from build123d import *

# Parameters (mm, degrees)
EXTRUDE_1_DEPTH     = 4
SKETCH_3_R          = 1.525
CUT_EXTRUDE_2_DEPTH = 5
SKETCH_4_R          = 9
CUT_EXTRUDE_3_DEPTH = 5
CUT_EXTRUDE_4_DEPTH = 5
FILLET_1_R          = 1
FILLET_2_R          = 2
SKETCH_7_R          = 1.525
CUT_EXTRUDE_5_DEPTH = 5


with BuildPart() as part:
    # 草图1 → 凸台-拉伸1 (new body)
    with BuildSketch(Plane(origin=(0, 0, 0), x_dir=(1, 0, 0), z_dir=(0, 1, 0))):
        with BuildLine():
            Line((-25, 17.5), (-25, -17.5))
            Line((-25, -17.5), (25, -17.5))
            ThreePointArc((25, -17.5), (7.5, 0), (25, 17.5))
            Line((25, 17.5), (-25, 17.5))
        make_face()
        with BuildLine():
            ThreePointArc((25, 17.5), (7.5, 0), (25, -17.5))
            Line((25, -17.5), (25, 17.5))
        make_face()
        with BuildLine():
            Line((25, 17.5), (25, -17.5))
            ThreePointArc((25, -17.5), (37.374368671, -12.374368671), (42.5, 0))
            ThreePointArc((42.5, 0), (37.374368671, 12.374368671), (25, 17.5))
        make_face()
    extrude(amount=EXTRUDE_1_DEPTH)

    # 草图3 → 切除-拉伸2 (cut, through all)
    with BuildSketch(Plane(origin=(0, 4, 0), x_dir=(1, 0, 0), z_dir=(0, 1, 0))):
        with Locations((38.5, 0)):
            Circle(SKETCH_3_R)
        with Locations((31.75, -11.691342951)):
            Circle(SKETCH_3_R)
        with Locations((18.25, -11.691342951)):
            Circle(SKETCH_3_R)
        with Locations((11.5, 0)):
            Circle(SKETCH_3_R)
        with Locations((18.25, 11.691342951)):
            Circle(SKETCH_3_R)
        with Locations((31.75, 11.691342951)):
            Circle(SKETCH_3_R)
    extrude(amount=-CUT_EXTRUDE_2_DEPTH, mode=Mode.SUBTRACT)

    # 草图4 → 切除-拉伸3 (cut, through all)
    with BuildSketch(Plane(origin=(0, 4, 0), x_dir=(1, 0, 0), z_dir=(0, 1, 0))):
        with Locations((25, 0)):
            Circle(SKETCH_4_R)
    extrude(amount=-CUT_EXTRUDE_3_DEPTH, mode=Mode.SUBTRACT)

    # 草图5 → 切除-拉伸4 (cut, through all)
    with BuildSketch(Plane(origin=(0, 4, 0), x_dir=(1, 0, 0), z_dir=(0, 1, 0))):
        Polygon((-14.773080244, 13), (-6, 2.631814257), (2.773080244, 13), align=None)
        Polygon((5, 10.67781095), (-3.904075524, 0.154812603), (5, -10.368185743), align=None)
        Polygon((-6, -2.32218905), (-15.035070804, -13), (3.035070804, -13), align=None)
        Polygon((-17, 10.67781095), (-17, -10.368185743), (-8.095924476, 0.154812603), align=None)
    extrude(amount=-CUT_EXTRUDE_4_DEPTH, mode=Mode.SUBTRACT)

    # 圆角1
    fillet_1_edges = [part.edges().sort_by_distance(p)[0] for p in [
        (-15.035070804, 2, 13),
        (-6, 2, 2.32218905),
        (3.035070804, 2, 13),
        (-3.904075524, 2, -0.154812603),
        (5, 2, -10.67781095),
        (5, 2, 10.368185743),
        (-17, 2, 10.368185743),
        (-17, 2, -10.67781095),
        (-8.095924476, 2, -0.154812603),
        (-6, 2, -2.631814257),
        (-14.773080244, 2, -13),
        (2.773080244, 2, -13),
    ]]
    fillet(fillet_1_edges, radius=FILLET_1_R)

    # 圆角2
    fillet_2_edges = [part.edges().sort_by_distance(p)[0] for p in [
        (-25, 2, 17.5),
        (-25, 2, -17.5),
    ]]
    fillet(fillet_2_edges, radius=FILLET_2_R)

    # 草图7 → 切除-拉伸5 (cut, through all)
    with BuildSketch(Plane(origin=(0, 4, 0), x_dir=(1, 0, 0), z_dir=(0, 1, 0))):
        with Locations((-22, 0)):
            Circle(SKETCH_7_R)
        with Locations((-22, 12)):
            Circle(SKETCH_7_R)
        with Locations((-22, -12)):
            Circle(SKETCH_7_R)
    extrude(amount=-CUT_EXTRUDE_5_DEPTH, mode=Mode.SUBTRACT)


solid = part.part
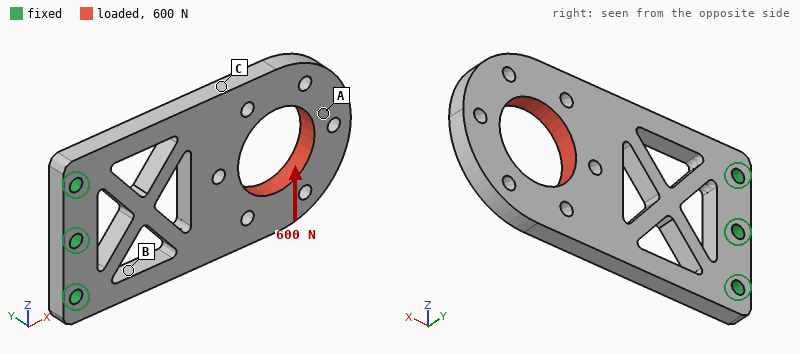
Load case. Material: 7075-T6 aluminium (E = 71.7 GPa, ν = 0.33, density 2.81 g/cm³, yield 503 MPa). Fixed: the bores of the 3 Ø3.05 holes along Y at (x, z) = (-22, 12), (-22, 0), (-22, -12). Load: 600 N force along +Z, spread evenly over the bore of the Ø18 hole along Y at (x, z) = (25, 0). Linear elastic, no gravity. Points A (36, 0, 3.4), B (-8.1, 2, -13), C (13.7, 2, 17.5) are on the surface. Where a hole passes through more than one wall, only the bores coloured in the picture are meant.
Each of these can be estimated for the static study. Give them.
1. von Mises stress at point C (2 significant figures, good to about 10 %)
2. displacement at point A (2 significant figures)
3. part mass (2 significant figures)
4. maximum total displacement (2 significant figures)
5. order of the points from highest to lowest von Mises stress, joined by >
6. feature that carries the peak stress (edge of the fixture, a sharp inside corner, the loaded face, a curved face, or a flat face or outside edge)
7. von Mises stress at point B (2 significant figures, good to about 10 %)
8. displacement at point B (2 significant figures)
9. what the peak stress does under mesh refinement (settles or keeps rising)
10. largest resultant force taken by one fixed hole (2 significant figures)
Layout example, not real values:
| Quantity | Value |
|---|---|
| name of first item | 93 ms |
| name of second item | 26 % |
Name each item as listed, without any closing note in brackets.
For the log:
| Quantity | Value |
|---|---|
| von Mises stress at point C | 20 MPa |
| displacement at point A | 82 µm |
| part mass | 17 g |
| maximum total displacement | 88 µm |
| order of the points from highest to lowest von Mises stress, joined by > | B > C > A |
| feature that carries the peak stress | edge of the fixture |
| von Mises stress at point B | 34 MPa |
| displacement at point B | 17 µm |
| what the peak stress does under mesh refinement | keeps rising |
| largest resultant force taken by one fixed hole | 1.0 kN |
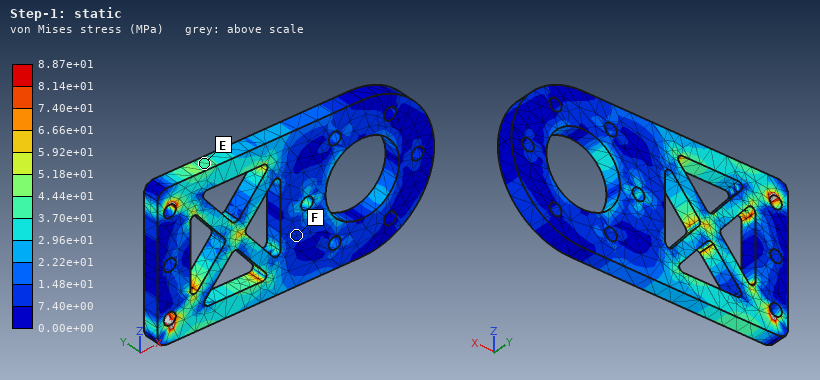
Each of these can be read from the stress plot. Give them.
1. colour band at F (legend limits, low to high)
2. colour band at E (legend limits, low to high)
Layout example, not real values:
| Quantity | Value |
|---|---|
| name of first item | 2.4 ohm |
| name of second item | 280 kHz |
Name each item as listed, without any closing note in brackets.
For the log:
| Quantity | Value |
|---|---|
| colour band at F | 7.40e+00 to 1.48e+01 MPa |
| colour band at E | 3.70e+01 to 4.44e+01 MPa |
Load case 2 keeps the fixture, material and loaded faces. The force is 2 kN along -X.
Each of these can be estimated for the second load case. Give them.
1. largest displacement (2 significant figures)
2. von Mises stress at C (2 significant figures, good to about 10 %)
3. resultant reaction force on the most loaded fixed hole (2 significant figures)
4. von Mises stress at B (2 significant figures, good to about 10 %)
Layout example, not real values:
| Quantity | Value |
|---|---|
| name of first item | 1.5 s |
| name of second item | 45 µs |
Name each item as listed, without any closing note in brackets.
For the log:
| Quantity | Value |
|---|---|
| largest displacement | 33 µm |
| von Mises stress at C | 42 MPa |
| resultant reaction force on the most loaded fixed hole | 1.1 kN |
| von Mises stress at B | 64 MPa |
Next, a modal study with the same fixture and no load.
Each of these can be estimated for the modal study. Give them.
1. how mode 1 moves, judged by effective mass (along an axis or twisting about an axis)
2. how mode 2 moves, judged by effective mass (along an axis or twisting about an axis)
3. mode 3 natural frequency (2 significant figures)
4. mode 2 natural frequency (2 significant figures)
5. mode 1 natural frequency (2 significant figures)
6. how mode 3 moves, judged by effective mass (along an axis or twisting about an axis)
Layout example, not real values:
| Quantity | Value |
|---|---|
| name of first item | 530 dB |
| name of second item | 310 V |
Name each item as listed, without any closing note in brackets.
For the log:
| Quantity | Value |
|---|---|
| how mode 1 moves, judged by effective mass | along Y |
| how mode 2 moves, judged by effective mass | twisting about X |
| mode 3 natural frequency | 4300 Hz |
| mode 2 natural frequency | 2700 Hz |
| mode 1 natural frequency | 690 Hz |
| how mode 3 moves, judged by effective mass | along Y |
